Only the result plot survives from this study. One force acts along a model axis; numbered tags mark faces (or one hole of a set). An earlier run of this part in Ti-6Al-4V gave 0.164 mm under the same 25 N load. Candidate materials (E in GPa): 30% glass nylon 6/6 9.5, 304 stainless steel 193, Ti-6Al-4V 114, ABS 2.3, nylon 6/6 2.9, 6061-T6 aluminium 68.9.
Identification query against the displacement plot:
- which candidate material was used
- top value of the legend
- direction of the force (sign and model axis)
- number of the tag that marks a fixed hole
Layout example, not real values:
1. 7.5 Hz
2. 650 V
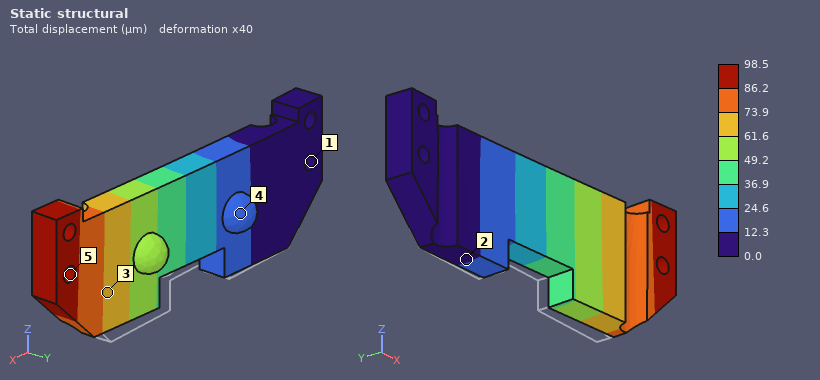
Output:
1. 304 stainless steel
2. 98.5 µm
3. -Y
4. 1
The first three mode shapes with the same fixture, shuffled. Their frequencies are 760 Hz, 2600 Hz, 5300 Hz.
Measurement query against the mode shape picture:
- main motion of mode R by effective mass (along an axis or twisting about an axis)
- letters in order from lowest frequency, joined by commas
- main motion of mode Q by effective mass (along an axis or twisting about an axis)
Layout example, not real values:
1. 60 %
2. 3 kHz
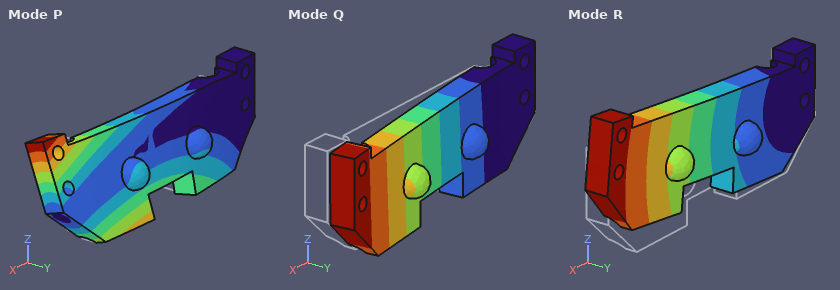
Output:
1. along Z
2. Q, R, P
3. along Y
